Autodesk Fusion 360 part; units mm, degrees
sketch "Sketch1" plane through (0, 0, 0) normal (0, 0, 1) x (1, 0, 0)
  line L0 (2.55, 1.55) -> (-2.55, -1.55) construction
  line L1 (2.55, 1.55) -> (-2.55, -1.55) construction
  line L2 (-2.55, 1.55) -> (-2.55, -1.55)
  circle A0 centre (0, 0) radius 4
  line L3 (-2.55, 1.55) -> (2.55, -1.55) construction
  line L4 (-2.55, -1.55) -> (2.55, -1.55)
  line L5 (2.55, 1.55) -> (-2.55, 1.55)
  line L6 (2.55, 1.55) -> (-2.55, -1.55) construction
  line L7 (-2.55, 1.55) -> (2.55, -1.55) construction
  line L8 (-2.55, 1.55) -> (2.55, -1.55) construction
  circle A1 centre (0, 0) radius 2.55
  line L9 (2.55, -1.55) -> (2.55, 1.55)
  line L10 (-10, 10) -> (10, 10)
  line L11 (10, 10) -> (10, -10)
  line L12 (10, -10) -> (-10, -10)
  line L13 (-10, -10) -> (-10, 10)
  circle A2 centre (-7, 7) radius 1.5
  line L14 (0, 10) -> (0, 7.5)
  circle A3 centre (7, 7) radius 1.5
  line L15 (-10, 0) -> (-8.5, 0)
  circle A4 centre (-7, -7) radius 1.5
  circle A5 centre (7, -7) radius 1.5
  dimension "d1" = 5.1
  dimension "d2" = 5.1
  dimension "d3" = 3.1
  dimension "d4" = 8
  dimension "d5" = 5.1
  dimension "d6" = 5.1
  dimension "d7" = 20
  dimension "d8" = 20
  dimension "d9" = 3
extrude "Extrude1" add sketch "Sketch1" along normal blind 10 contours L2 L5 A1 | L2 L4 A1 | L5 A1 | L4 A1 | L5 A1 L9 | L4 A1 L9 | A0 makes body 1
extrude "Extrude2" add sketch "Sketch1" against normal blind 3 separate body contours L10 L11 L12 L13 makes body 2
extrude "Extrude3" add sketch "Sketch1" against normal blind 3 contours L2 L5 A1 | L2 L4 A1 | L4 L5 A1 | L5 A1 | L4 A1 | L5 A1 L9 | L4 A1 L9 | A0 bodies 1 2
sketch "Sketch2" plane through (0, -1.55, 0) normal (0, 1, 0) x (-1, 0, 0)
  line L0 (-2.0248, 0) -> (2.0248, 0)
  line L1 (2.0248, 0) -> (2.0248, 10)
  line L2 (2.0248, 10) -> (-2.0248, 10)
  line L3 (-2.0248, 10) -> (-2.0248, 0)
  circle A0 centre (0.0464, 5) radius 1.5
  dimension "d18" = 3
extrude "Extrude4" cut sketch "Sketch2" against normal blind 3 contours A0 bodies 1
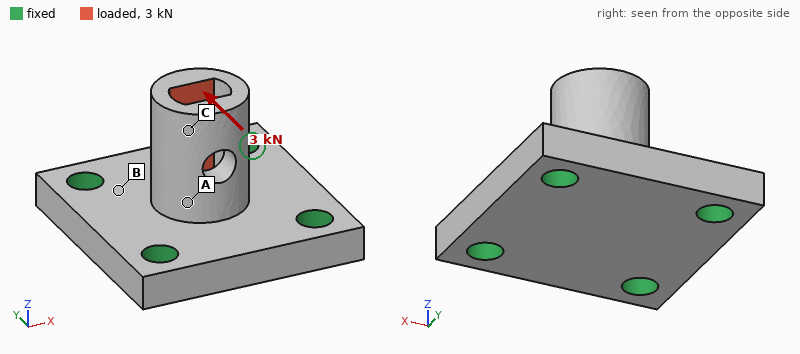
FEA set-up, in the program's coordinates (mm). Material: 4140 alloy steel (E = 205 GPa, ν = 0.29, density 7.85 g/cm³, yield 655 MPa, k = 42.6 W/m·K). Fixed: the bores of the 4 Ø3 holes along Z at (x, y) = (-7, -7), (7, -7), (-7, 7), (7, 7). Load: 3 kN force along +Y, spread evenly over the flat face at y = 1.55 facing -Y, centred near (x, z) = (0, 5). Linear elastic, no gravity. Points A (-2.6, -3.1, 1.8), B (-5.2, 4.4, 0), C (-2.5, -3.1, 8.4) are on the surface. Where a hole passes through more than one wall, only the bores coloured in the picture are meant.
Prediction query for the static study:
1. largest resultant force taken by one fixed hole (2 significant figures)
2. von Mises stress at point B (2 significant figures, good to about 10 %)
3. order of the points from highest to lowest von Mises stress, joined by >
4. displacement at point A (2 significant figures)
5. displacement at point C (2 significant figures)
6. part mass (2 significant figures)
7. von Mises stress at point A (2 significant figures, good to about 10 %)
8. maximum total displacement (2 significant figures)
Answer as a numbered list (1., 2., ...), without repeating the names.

1. 1.2 kN
2. 110 MPa
3. A > B > C
4. 13 µm
5. 40 µm
6. 11 g
7. 250 MPa
8. 52 µm
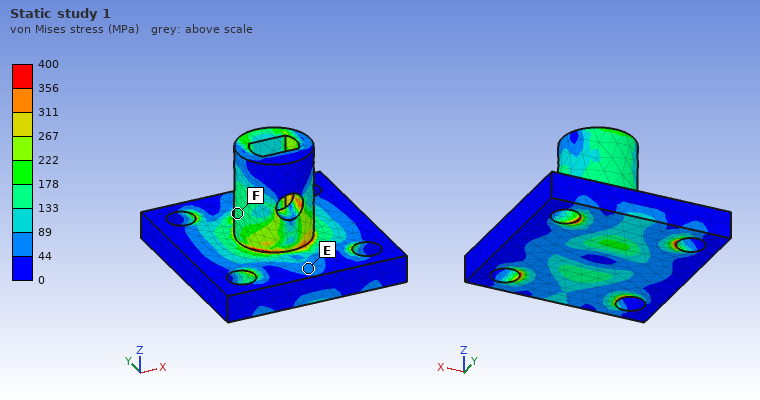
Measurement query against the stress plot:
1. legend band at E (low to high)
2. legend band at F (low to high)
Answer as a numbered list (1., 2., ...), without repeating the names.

1. 44 to 89 MPa
2. 133 to 178 MPa
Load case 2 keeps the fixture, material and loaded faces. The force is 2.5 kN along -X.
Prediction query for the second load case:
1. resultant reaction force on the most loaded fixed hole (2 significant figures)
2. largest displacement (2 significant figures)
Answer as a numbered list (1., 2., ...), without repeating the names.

1. 1.1 kN
2. 42 µm
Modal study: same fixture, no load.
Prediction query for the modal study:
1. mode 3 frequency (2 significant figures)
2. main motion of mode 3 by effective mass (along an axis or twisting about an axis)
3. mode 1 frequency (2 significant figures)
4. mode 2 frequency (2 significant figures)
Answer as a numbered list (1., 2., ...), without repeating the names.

1. 43 kHz
2. along Z
3. 29 kHz
4. 29 kHz
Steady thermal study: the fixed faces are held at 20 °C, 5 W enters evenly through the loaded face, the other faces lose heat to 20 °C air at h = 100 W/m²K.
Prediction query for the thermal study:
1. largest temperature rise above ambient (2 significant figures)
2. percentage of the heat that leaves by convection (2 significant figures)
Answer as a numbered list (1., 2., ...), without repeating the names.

1. 31 K
2. 18 %
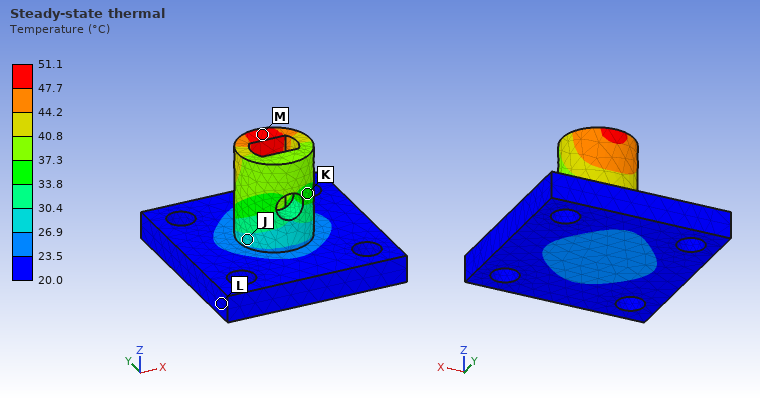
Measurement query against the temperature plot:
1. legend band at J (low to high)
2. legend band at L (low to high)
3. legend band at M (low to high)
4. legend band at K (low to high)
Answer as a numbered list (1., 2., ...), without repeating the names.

1. 26.9 to 30.4 °C
2. 20.0 to 23.5 °C
3. 47.7 to 51.1 °C
4. 33.8 to 37.3 °C
